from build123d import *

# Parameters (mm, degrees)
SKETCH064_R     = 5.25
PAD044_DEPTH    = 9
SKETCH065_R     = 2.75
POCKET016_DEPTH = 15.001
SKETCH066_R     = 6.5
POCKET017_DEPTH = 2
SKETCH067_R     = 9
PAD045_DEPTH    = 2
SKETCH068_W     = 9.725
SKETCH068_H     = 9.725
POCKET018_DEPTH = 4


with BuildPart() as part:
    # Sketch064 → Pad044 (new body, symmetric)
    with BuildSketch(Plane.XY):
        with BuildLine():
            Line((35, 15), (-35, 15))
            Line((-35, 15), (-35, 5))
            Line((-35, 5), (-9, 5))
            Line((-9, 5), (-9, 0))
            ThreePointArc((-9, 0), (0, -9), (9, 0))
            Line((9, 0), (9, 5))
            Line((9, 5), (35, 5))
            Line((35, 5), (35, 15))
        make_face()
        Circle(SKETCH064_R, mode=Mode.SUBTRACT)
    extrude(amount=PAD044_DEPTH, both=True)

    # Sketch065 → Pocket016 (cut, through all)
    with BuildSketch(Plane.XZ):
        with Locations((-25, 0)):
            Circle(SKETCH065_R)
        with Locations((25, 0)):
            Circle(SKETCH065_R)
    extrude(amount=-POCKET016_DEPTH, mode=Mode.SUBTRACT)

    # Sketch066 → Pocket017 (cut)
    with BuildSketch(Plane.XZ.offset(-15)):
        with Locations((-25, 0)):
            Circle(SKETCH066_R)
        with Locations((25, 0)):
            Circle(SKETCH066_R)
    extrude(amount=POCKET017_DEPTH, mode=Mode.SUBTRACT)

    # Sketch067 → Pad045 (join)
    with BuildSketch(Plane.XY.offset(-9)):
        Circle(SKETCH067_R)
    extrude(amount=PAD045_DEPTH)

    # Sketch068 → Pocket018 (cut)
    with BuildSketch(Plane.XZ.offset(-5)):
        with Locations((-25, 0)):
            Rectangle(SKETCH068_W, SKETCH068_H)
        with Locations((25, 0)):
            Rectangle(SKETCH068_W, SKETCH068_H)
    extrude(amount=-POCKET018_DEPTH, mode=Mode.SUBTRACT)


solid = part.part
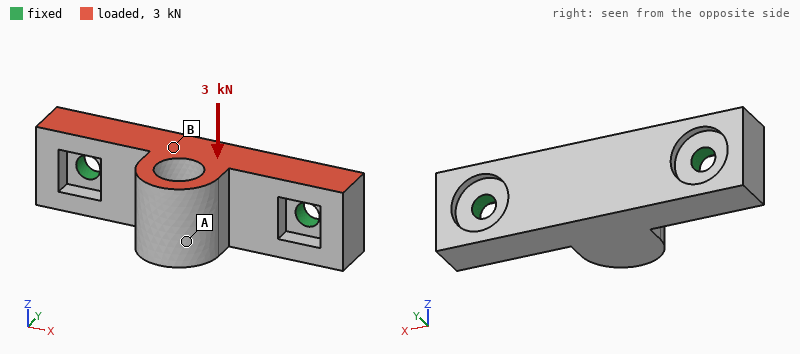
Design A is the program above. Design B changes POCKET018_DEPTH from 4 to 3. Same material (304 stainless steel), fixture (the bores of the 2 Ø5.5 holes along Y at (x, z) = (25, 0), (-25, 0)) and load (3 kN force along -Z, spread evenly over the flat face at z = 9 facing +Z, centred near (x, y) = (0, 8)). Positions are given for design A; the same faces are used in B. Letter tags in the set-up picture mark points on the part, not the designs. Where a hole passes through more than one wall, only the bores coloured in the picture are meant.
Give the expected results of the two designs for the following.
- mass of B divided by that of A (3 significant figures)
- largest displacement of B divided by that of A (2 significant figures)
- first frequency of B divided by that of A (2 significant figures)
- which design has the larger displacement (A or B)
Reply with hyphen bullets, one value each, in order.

- 1.01
- 0.76
- 1.1
- A
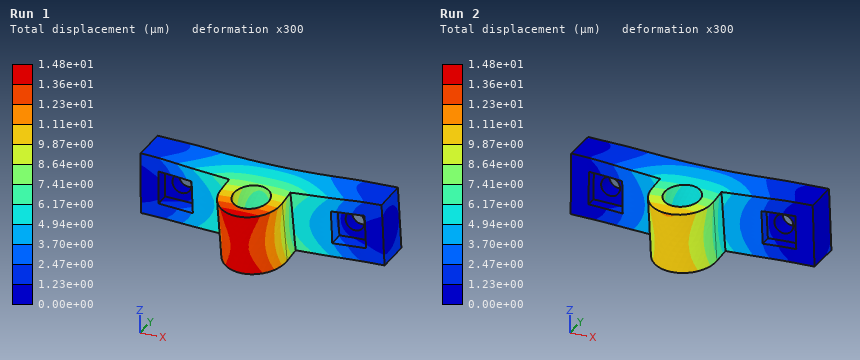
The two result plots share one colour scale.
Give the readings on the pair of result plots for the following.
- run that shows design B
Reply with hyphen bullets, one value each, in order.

- Run 2
